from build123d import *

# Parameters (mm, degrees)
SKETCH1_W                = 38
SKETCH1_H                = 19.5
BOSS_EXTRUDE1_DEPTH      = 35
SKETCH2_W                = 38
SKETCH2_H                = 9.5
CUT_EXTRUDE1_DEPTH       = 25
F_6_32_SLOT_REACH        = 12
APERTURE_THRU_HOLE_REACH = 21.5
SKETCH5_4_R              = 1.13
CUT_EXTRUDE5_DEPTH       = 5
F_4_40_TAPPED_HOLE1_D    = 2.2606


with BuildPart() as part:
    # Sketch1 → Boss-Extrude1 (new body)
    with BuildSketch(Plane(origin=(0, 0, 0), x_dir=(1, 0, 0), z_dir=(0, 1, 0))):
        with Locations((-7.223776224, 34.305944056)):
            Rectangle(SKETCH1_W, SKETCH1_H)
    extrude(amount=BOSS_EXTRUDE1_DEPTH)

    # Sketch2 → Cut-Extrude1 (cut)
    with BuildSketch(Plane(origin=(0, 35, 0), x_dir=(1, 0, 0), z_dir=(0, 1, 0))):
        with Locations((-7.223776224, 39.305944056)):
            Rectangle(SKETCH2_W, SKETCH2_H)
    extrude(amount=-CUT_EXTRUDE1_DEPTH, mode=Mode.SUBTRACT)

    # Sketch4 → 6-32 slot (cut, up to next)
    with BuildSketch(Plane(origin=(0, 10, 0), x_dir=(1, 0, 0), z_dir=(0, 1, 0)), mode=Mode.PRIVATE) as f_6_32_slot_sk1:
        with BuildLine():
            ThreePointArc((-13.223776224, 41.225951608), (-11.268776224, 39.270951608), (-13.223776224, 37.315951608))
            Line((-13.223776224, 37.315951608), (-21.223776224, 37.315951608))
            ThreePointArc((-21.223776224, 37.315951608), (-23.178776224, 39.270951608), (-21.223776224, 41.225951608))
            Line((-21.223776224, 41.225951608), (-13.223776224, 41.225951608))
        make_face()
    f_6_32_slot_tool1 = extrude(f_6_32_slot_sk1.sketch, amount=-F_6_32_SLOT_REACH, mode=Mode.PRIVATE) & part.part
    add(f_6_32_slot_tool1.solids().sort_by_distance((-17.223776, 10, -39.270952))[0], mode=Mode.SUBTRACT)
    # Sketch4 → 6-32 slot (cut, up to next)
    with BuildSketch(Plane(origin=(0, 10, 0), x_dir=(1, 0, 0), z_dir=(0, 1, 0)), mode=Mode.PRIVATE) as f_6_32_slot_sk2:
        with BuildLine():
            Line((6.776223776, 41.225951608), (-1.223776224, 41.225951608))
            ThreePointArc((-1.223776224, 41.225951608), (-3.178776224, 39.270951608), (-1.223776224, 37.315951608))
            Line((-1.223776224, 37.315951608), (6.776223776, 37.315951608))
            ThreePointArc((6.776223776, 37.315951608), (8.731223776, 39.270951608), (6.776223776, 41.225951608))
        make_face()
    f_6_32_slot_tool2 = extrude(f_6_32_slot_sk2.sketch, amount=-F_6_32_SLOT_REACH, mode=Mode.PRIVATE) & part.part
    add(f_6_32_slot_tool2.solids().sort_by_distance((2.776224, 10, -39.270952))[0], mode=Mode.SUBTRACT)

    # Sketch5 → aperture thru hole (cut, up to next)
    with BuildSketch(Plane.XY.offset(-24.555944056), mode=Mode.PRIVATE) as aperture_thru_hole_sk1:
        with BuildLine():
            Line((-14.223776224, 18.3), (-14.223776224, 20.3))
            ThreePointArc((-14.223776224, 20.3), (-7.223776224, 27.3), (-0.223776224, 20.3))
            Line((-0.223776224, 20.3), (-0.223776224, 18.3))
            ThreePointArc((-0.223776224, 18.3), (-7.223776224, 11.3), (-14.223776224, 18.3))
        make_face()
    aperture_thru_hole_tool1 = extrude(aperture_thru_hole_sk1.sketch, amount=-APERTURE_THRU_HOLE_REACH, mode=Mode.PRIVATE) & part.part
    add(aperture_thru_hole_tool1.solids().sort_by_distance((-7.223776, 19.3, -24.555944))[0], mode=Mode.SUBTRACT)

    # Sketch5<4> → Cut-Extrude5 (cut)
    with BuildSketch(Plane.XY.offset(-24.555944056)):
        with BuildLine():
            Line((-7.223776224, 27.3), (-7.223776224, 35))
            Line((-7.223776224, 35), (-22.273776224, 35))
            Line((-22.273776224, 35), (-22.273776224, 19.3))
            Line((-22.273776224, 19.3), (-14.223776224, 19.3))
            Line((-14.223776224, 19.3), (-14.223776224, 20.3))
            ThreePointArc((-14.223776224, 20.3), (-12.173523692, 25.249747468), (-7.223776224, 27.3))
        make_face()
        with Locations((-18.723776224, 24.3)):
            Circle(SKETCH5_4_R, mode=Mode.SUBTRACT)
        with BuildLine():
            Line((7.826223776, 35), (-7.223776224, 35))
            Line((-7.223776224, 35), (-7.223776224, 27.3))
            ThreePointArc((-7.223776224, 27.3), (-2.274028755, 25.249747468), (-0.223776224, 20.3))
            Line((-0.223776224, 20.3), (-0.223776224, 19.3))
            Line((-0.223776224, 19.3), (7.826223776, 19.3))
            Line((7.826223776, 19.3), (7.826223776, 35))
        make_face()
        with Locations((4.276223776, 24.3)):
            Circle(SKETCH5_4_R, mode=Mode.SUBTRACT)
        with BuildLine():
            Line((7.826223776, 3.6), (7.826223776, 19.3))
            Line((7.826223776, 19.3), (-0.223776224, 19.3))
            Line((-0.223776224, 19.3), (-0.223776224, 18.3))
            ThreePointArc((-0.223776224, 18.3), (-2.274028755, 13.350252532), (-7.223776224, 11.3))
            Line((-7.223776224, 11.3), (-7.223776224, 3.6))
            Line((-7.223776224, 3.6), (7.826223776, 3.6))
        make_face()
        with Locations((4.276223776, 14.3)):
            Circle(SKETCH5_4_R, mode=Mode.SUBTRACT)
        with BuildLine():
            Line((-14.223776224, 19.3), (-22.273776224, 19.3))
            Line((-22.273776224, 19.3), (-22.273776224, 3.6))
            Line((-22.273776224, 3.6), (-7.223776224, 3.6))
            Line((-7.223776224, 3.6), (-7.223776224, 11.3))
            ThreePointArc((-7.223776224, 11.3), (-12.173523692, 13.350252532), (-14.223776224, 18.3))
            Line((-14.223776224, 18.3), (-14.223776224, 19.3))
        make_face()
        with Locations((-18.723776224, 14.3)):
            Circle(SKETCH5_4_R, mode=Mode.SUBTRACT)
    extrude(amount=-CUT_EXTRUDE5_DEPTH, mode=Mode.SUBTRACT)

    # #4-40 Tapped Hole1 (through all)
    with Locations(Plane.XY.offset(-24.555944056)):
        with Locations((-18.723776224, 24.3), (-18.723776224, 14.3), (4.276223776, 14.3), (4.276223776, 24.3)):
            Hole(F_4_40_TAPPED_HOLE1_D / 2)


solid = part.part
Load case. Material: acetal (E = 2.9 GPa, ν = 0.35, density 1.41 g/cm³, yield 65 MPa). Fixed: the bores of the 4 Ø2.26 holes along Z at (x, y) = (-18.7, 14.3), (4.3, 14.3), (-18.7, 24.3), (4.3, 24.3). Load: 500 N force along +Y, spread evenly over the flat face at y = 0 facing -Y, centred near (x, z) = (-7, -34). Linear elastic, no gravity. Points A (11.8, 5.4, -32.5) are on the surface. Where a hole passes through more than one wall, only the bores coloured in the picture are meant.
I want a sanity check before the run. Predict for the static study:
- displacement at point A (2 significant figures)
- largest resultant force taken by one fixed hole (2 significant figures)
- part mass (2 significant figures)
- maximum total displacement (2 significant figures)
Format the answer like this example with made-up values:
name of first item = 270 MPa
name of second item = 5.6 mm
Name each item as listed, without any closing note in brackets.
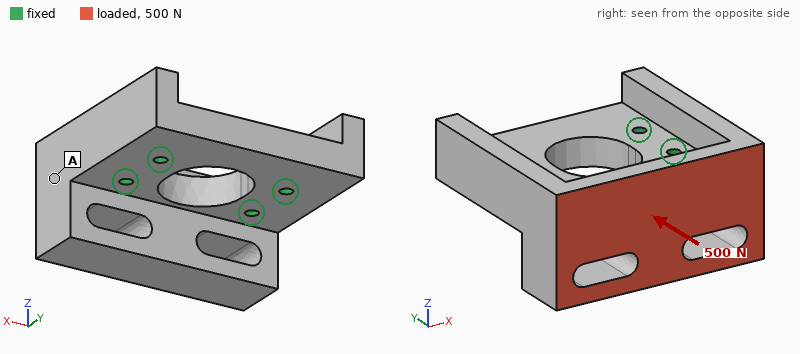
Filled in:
displacement at point A = 0.031 mm
largest resultant force taken by one fixed hole = 210 N
part mass = 15 g
maximum total displacement = 0.10 mm
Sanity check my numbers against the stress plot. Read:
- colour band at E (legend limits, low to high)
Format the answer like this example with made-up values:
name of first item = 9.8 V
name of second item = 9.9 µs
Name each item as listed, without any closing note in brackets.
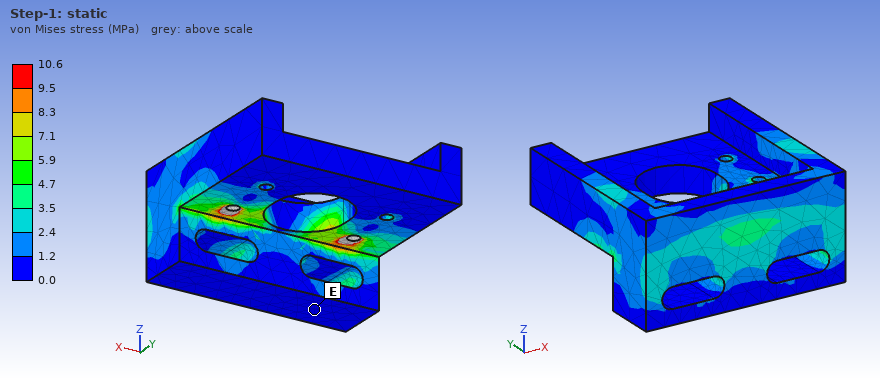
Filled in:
colour band at E = 0.0 to 1.2 MPa
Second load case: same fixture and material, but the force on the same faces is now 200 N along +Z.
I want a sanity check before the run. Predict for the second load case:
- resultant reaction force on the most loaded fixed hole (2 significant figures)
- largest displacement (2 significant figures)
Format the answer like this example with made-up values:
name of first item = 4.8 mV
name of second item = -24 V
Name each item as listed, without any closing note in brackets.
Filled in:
resultant reaction force on the most loaded fixed hole = 170 N
largest displacement = 0.21 mm
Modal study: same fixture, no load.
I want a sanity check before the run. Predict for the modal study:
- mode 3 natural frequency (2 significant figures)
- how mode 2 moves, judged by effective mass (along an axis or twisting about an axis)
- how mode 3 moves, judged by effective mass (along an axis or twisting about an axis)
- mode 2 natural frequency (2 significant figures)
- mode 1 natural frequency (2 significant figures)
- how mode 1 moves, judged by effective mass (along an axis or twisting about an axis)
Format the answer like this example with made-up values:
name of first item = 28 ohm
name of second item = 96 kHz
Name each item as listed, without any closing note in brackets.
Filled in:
mode 3 natural frequency = 6100 Hz
how mode 2 moves, judged by effective mass = twisting about Y
how mode 3 moves, judged by effective mass = along X
mode 2 natural frequency = 4000 Hz
mode 1 natural frequency = 2500 Hz
how mode 1 moves, judged by effective mass = along Z
